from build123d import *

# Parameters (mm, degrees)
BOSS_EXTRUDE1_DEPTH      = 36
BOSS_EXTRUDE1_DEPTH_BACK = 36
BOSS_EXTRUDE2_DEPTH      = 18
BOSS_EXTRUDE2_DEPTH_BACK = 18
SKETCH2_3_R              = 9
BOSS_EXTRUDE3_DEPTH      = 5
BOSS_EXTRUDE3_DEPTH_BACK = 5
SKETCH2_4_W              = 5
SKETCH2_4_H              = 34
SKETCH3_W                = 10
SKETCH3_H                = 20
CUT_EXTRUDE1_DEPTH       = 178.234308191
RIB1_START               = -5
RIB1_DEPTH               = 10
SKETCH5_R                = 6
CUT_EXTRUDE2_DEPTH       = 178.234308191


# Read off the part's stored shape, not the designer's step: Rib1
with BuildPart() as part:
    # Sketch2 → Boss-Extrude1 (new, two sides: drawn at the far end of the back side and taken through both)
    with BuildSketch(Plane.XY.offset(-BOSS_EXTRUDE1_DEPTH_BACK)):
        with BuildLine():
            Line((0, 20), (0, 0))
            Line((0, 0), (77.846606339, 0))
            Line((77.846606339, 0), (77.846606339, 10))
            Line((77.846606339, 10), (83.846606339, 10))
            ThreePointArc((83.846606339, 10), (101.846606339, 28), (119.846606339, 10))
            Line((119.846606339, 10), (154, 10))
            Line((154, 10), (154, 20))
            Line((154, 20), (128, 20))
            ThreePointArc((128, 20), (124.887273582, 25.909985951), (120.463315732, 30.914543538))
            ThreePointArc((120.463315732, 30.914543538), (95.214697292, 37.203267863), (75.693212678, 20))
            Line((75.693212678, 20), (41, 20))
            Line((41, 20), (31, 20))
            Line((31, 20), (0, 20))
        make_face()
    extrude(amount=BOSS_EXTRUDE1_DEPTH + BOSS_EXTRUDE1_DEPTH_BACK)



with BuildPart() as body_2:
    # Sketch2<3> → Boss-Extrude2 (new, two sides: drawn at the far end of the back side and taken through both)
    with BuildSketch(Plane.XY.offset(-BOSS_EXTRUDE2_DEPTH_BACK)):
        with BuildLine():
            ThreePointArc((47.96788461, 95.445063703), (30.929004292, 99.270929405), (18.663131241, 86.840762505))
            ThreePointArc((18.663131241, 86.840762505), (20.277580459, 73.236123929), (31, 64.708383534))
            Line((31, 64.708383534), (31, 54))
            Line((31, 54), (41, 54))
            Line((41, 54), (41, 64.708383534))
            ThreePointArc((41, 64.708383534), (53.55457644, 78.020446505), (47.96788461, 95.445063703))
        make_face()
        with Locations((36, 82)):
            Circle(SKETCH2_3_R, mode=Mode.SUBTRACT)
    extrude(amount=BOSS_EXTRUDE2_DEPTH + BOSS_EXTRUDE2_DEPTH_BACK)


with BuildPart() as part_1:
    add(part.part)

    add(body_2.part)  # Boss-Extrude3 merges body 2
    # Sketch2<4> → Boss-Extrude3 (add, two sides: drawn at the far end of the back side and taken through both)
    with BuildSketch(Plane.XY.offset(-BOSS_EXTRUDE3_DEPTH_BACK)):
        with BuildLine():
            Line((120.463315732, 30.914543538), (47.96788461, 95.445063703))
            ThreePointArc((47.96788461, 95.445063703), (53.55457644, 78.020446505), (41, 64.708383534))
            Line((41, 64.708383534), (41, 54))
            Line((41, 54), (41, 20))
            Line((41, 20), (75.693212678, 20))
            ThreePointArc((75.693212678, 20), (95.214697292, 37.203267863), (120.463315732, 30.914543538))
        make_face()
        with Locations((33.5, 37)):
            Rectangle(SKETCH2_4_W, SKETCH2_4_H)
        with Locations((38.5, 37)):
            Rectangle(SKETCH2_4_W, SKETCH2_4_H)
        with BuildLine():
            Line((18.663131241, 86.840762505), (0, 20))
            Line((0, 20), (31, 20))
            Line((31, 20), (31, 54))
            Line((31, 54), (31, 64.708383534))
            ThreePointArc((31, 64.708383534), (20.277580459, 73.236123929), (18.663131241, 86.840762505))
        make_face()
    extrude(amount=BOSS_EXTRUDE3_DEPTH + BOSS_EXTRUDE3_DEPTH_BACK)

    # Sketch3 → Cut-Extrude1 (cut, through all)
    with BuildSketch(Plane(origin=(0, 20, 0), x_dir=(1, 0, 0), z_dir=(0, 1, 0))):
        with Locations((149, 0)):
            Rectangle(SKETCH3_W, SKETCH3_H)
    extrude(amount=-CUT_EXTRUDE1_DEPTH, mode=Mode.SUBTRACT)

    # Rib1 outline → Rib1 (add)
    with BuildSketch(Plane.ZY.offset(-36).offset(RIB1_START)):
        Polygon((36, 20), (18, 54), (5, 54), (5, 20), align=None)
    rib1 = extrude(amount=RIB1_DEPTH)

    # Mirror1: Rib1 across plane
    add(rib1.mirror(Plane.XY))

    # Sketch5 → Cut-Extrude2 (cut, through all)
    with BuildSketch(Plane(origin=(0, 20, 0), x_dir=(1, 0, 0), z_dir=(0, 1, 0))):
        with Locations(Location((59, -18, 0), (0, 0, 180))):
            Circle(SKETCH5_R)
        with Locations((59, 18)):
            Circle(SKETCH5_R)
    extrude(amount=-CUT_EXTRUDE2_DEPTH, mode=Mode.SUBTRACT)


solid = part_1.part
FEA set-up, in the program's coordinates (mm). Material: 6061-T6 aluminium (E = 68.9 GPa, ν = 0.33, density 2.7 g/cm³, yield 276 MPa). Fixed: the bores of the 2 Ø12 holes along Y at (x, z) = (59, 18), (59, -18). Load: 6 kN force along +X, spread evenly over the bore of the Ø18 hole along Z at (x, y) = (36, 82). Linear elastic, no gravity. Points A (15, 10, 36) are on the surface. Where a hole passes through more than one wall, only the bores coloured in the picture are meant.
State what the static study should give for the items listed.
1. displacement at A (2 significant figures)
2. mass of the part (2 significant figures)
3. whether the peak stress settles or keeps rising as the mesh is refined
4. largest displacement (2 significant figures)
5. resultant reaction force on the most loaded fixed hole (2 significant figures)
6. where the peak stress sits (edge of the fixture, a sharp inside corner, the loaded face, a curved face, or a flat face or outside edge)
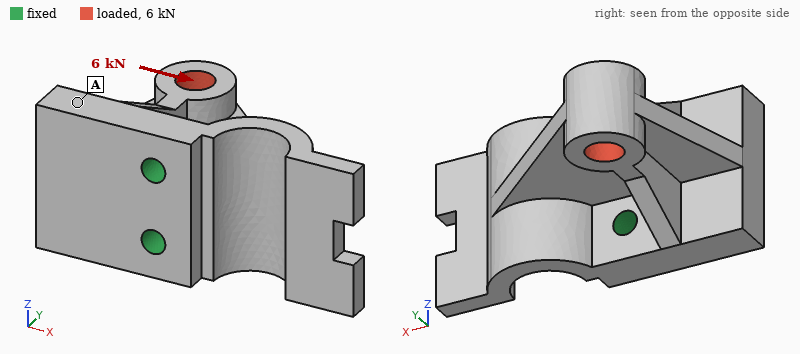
0.043 mm
710 g
keeps rising
0.14 mm
3.0 kN
edge of the fixture
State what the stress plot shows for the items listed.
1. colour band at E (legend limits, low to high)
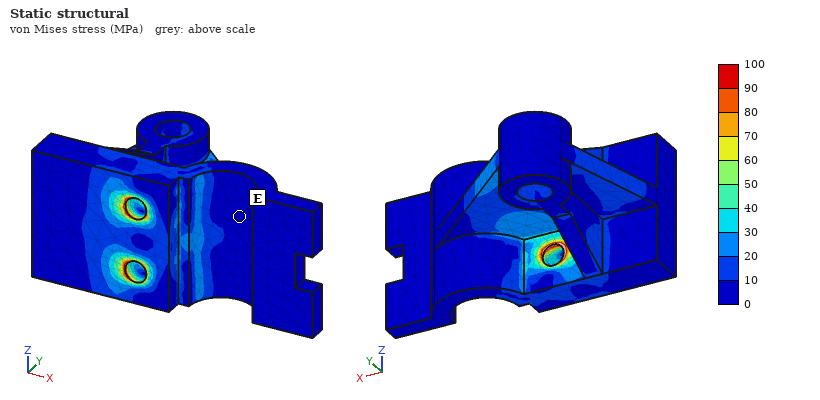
0 to 10 MPa
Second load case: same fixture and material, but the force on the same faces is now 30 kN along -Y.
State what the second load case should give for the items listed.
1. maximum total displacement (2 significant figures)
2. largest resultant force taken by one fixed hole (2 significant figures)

0.19 mm
15 kN
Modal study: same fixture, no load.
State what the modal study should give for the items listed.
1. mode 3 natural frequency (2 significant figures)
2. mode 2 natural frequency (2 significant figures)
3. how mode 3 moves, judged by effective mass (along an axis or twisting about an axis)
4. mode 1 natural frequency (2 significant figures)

3100 Hz
2300 Hz
along X
1800 Hz
